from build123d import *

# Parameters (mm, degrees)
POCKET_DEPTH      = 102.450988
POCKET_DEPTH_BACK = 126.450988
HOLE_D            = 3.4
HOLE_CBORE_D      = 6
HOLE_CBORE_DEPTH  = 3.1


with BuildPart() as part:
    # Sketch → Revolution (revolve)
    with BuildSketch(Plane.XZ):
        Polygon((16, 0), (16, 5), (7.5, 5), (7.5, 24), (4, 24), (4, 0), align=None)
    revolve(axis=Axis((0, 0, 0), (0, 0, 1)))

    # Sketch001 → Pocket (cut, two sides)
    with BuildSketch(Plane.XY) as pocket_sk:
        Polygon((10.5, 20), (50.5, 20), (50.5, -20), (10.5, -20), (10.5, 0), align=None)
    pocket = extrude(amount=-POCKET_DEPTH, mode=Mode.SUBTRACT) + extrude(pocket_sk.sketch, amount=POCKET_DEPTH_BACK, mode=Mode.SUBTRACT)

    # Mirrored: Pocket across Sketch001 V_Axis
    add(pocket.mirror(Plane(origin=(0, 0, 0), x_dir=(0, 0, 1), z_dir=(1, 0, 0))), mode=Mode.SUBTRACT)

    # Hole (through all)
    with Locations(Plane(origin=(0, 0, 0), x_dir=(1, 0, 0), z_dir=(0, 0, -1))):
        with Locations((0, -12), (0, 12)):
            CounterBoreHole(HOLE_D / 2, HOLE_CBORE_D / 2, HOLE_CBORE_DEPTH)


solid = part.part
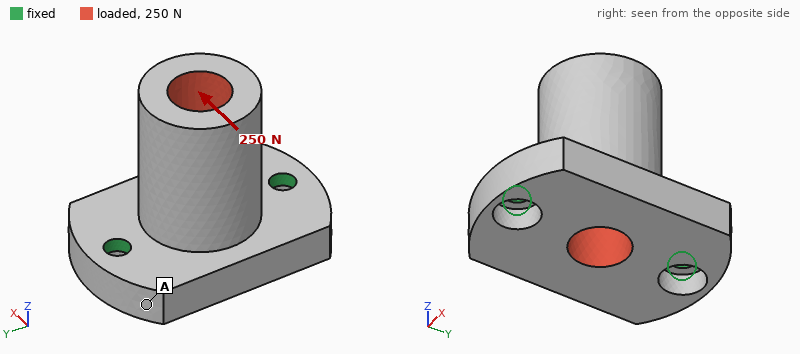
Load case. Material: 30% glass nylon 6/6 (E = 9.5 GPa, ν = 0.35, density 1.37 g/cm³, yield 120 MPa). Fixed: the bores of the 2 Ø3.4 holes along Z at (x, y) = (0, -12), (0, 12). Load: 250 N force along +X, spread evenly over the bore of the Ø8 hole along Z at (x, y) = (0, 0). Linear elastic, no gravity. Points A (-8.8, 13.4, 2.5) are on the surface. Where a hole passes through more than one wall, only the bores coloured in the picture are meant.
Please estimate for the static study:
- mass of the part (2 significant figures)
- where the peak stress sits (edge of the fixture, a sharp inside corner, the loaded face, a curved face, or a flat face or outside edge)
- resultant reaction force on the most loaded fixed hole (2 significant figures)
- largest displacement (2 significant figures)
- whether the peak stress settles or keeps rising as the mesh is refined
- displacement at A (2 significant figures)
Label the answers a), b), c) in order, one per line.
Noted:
a) 6.9 g
b) edge of the fixture
c) 130 N
d) 0.25 mm
e) keeps rising
f) 0.072 mm
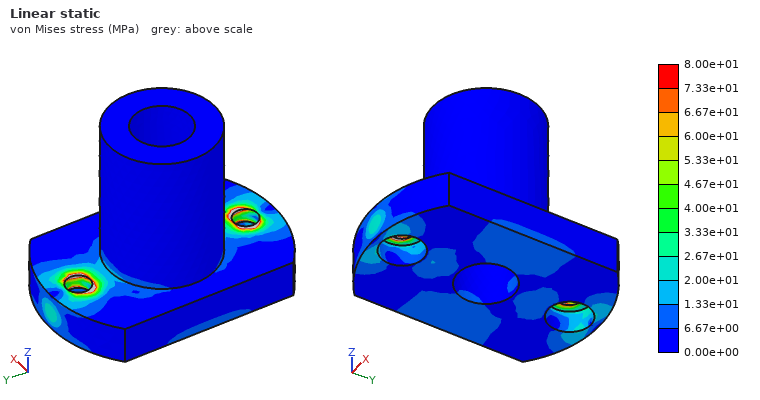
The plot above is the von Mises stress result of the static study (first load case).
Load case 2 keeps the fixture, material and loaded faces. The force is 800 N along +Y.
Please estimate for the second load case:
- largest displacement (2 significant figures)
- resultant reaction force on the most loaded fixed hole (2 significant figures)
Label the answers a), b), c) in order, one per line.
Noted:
a) 0.13 mm
b) 500 N
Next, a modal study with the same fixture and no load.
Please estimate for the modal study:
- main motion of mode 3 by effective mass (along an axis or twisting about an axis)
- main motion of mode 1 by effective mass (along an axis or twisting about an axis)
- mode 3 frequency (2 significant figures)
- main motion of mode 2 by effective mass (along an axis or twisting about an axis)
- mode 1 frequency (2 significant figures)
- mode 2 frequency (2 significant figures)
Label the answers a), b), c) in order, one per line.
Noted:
a) along Z
b) along X
c) 8400 Hz
d) along Y
e) 2600 Hz
f) 7100 Hz
